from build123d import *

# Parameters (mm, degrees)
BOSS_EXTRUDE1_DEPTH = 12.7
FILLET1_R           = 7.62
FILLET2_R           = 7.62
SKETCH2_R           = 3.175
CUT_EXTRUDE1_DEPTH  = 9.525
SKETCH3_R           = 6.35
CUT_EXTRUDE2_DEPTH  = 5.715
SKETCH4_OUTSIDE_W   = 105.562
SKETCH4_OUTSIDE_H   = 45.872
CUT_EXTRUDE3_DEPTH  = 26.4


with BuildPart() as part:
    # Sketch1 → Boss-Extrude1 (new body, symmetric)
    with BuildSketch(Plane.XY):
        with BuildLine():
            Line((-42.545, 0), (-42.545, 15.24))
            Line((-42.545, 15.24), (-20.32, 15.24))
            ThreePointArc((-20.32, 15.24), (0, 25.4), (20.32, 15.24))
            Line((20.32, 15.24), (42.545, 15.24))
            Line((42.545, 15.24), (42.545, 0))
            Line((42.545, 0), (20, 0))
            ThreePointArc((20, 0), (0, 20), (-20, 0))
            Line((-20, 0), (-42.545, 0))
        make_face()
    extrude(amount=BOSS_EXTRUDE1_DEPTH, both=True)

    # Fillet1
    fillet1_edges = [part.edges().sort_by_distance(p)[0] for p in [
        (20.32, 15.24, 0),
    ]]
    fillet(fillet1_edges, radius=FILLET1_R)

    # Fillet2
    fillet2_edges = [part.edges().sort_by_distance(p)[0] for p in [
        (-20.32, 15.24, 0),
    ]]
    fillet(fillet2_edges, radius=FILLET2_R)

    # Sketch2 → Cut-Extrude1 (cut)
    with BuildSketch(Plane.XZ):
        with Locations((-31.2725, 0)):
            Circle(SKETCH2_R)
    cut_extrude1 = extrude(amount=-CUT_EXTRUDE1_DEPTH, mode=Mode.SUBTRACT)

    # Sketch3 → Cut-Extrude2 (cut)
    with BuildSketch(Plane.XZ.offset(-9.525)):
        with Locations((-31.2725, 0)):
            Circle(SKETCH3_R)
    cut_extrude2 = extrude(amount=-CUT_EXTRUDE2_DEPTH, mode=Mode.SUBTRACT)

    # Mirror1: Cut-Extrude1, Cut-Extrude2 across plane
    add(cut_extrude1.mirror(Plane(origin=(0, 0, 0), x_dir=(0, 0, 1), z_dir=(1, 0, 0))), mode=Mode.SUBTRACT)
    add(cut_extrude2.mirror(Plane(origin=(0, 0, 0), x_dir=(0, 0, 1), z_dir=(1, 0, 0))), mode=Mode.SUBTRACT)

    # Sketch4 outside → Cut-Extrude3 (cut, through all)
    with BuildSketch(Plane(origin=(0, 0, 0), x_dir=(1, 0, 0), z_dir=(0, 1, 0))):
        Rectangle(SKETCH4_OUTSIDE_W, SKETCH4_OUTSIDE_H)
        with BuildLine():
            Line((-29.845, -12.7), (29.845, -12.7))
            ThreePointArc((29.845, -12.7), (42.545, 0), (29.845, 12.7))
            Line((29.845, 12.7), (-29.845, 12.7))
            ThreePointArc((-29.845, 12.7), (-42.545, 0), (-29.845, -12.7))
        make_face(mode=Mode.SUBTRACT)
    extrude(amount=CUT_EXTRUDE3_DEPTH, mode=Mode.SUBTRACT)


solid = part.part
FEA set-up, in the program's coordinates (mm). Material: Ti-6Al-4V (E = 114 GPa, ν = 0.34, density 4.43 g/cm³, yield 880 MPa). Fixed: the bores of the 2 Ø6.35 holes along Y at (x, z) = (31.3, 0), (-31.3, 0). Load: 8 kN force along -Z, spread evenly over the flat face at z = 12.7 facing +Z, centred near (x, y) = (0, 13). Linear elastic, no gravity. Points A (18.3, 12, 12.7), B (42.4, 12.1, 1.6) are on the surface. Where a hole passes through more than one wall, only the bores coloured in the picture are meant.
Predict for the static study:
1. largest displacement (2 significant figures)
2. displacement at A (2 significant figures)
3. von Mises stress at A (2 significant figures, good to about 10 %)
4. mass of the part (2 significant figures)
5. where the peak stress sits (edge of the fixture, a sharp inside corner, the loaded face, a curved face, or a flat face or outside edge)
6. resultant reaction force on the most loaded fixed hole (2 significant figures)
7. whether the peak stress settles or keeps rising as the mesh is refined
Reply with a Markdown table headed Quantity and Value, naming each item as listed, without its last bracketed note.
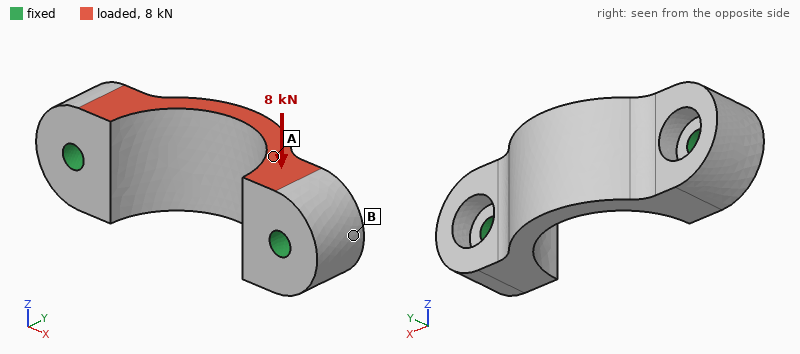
| Quantity | Value |
|---|---|
| largest displacement | 51 µm |
| displacement at A | 24 µm |
| von Mises stress at A | 33 MPa |
| mass of the part | 90 g |
| where the peak stress sits | edge of the fixture |
| resultant reaction force on the most loaded fixed hole | 4.0 kN |
| whether the peak stress settles or keeps rising as the mesh is refined | keeps rising |
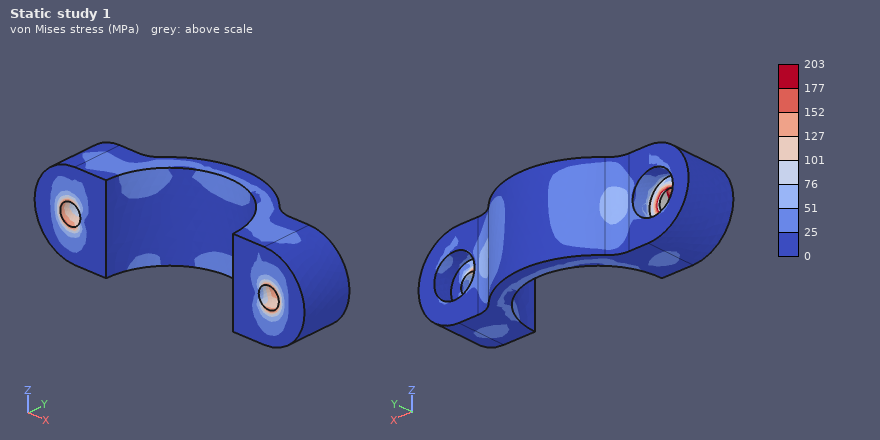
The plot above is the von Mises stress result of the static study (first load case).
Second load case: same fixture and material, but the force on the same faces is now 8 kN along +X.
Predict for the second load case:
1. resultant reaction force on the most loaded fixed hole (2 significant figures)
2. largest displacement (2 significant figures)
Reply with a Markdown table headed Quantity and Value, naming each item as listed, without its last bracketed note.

| Quantity | Value |
|---|---|
| resultant reaction force on the most loaded fixed hole | 4.2 kN |
| largest displacement | 25 µm |
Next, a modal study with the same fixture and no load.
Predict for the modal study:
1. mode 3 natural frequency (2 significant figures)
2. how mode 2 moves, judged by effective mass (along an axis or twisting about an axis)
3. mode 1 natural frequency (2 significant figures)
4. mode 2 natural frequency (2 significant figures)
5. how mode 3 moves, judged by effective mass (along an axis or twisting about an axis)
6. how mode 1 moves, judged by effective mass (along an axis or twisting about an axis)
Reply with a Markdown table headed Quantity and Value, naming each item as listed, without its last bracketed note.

| Quantity | Value |
|---|---|
| mode 3 natural frequency | 20 kHz |
| how mode 2 moves, judged by effective mass | along X |
| mode 1 natural frequency | 9800 Hz |
| mode 2 natural frequency | 16 kHz |
| how mode 3 moves, judged by effective mass | along Y |
| how mode 1 moves, judged by effective mass | along Z |
